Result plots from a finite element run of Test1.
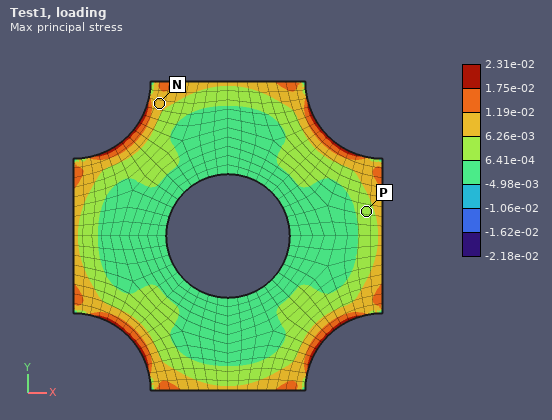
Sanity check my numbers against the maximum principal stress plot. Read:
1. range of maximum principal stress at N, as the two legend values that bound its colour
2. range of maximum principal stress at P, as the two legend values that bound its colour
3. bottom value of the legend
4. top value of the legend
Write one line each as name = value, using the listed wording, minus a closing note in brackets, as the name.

range of maximum principal stress at N, as the two legend values that bound its colour = 6.26e-03 to 1.19e-02
range of maximum principal stress at P, as the two legend values that bound its colour = 6.41e-04 to 6.26e-03
bottom value of the legend = -2.18e-02
top value of the legend = 2.31e-02
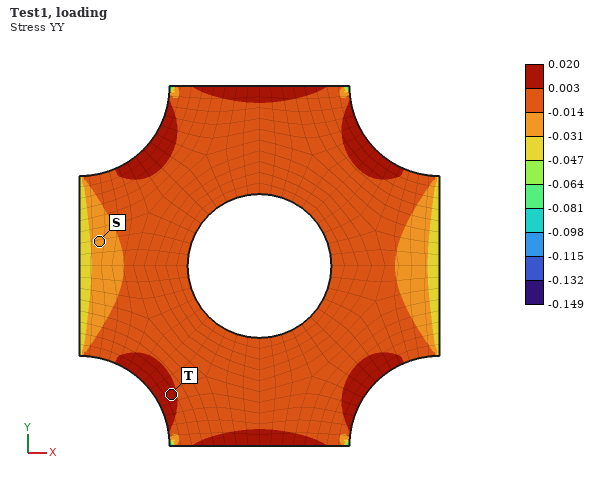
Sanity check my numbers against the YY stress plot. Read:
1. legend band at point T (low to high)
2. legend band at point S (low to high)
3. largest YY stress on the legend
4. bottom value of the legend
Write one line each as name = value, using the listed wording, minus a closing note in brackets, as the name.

legend band at point T = 0.003 to 0.020
legend band at point S = -0.031 to -0.014
largest YY stress on the legend = 0.020
bottom value of the legend = -0.149
